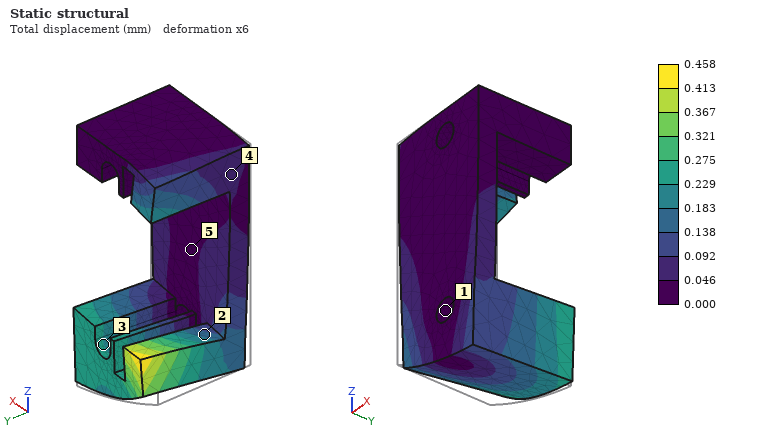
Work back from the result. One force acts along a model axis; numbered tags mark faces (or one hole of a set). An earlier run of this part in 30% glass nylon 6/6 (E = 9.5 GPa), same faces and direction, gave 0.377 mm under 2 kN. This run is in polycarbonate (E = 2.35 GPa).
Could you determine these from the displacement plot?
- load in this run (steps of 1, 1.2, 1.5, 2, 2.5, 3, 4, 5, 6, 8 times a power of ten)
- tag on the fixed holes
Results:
600 N
1
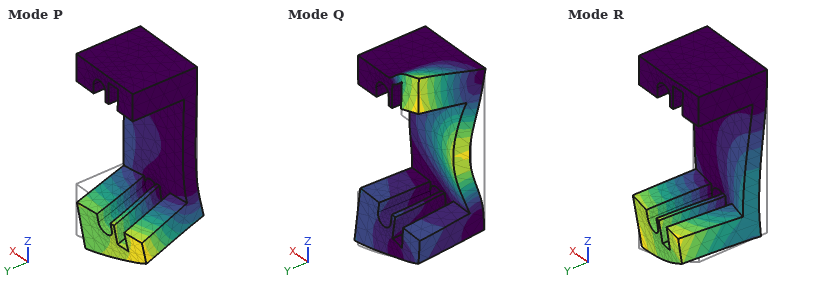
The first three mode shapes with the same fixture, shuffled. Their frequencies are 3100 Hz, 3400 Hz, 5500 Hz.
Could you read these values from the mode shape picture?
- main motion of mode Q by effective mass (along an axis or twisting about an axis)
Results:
along Y
